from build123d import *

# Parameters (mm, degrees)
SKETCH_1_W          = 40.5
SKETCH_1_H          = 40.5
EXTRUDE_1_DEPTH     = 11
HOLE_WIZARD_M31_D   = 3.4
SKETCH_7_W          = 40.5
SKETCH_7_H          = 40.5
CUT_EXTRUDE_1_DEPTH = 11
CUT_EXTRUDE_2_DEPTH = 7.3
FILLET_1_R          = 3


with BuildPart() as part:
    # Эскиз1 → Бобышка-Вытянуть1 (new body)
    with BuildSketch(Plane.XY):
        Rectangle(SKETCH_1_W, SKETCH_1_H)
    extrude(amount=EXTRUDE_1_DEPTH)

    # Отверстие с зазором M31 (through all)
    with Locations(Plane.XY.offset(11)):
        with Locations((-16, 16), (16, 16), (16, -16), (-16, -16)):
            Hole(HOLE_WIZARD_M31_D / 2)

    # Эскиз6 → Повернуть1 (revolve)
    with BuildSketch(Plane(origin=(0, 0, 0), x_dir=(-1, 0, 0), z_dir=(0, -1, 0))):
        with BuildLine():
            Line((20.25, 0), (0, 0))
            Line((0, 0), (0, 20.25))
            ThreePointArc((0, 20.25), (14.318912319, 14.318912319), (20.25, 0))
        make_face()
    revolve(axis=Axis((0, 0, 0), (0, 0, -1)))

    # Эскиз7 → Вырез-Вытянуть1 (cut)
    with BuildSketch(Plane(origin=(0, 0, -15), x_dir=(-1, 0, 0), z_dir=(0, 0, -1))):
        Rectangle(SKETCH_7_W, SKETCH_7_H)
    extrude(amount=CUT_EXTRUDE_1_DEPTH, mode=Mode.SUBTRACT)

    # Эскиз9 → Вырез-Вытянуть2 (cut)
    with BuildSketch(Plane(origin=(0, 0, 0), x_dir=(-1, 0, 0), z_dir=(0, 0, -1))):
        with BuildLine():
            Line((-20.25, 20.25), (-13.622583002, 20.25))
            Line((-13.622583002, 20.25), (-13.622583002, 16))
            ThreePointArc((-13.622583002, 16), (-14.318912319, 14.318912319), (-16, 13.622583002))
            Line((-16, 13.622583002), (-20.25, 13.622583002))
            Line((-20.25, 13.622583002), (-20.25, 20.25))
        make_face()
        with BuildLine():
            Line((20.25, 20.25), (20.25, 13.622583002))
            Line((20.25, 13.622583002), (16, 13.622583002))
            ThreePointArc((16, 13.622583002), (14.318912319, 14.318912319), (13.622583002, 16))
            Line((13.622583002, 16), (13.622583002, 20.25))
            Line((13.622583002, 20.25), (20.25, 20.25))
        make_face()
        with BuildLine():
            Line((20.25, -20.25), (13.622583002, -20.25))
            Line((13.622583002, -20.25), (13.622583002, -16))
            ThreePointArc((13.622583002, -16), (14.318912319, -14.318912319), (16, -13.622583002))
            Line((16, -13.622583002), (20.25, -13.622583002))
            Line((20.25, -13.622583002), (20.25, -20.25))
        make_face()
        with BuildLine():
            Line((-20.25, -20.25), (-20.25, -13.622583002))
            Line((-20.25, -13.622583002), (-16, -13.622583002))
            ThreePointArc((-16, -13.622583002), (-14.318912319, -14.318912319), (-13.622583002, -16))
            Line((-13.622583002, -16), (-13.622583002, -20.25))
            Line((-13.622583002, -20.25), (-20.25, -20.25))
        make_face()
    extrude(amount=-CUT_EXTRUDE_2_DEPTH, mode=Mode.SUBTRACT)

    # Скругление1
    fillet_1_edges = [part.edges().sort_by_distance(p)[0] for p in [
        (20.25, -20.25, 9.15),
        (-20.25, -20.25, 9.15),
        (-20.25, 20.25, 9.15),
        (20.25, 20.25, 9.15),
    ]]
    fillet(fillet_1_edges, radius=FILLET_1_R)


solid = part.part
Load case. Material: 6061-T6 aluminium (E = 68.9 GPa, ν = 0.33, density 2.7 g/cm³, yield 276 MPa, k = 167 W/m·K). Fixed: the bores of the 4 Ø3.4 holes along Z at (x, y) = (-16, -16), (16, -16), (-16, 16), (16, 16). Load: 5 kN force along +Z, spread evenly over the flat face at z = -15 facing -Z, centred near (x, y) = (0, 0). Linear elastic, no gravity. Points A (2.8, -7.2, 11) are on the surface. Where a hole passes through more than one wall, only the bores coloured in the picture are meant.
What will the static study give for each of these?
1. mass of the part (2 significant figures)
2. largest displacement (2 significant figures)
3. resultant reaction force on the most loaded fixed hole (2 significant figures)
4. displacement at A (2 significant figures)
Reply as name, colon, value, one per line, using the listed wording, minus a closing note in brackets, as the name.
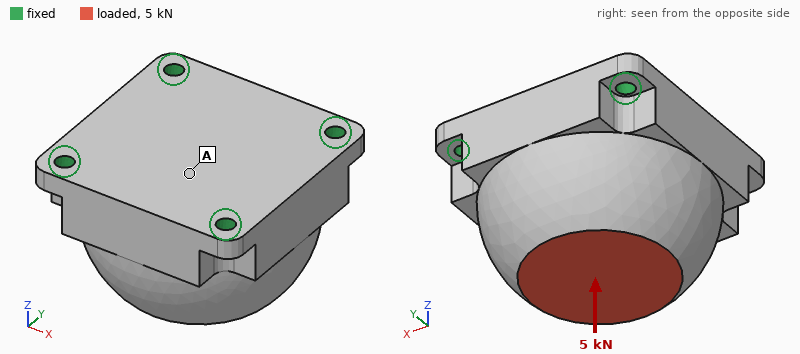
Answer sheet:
mass of the part: 88 g
largest displacement: 7.7 µm
resultant reaction force on the most loaded fixed hole: 1.4 kN
displacement at A: 6.1 µm
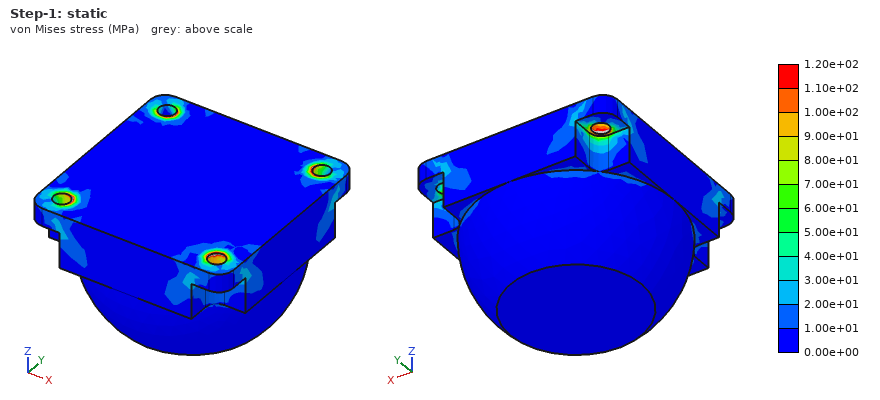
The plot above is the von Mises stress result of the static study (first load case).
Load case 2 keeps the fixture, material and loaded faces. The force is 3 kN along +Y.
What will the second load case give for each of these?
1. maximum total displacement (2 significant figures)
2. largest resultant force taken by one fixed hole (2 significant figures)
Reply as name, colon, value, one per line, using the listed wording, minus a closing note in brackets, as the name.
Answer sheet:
maximum total displacement: 13 µm
largest resultant force taken by one fixed hole: 1.4 kN
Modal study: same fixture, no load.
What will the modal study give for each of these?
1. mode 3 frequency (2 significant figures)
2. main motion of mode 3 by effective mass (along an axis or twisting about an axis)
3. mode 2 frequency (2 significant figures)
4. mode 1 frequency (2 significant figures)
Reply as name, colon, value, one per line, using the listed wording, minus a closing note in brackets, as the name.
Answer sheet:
mode 3 frequency: 16 kHz
main motion of mode 3 by effective mass: along Z
mode 2 frequency: 14 kHz
mode 1 frequency: 14 kHz
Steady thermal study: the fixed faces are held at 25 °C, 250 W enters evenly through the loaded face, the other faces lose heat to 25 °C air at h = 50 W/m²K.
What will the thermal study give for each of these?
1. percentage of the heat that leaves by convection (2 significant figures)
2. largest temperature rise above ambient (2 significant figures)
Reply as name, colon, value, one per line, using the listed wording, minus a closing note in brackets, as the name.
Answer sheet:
percentage of the heat that leaves by convection: 3.9 %
largest temperature rise above ambient: 70 K
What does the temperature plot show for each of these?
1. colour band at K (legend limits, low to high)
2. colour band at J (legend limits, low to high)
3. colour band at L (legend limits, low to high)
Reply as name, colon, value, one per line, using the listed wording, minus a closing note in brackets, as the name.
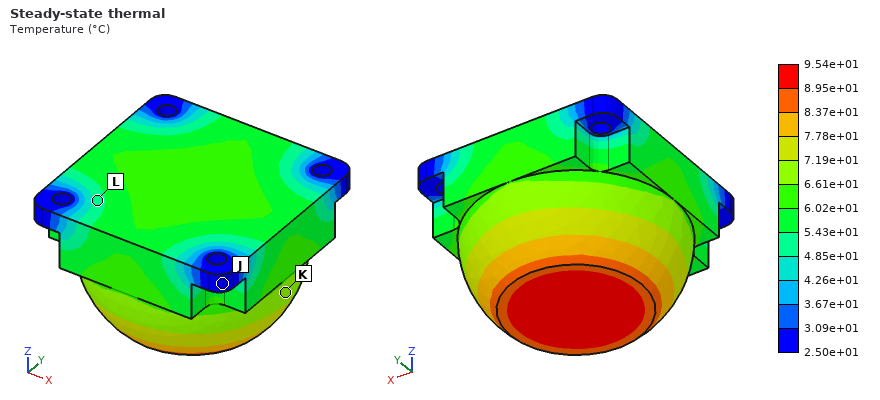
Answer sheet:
colour band at K: 6.61e+01 to 7.19e+01 °C
colour band at J: 2.50e+01 to 3.09e+01 °C
colour band at L: 4.85e+01 to 5.43e+01 °C
